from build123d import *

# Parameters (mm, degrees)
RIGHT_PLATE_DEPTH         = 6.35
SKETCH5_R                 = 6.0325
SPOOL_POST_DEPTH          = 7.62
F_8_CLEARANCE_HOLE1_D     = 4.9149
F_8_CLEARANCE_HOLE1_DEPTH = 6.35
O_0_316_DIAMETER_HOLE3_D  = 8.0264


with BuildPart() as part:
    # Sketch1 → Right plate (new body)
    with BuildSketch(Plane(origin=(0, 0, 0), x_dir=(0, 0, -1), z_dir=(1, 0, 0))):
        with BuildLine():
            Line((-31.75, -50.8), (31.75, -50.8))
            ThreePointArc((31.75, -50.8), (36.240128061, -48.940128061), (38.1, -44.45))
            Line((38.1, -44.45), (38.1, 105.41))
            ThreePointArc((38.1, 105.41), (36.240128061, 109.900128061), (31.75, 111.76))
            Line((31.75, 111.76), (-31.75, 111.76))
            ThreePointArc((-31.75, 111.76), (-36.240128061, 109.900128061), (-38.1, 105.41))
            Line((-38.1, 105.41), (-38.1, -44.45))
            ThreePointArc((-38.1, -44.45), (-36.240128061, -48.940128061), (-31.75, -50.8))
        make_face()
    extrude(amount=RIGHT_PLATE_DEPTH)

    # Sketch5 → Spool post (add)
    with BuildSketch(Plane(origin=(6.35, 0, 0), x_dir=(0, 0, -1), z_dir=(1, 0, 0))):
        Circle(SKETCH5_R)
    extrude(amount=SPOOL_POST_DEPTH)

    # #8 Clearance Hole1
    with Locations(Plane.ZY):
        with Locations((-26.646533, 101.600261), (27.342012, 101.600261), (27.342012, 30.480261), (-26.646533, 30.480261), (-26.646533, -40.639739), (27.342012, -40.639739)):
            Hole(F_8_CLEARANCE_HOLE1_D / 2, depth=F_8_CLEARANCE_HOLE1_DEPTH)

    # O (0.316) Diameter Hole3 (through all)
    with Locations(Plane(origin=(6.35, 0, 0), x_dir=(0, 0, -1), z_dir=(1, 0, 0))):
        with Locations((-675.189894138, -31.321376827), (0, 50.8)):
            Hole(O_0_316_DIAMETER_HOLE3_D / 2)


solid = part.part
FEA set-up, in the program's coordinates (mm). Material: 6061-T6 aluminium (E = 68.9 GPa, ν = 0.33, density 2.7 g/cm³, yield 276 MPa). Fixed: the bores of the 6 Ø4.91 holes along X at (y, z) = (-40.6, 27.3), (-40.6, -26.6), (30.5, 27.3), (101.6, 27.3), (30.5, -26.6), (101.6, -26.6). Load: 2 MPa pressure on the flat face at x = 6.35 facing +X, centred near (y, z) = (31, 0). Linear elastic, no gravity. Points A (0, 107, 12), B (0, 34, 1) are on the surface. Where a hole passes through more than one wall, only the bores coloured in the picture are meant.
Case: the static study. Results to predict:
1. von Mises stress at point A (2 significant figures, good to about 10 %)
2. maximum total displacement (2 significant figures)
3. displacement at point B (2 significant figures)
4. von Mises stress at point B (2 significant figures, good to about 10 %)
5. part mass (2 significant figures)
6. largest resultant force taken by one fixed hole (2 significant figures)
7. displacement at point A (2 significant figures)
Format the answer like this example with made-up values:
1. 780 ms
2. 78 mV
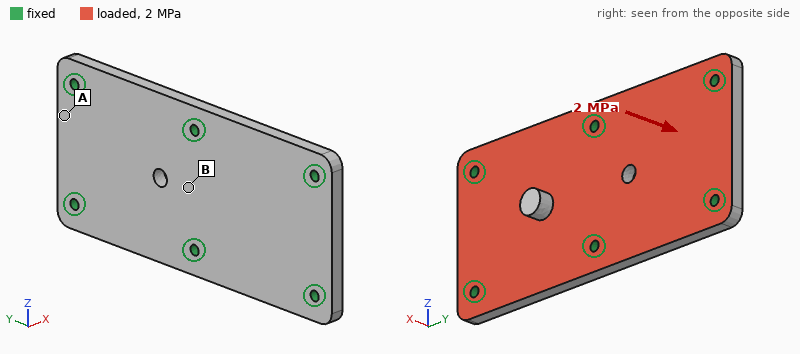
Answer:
1. 26 MPa
2. 0.14 mm
3. 0.074 mm
4. 75 MPa
5. 210 g
6. 5.5 kN
7. 0.023 mm
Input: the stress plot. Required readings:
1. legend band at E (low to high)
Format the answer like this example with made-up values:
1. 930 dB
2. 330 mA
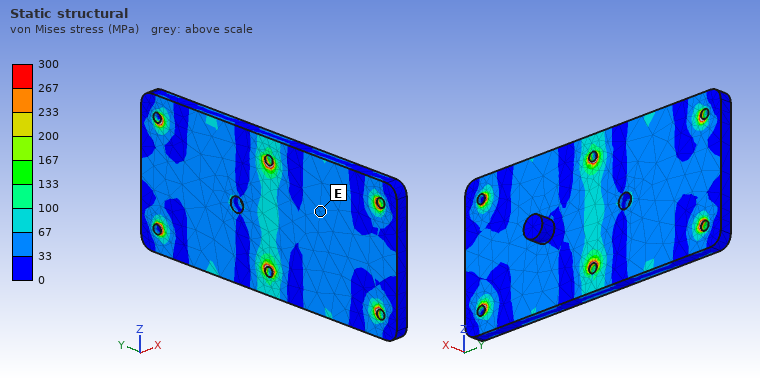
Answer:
1. 33 to 67 MPa
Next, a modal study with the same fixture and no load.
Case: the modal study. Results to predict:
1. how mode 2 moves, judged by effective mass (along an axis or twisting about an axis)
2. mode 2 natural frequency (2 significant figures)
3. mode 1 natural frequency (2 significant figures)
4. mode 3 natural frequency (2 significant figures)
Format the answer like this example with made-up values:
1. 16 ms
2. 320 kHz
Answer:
1. along X
2. 5400 Hz
3. 5000 Hz
4. 6900 Hz
